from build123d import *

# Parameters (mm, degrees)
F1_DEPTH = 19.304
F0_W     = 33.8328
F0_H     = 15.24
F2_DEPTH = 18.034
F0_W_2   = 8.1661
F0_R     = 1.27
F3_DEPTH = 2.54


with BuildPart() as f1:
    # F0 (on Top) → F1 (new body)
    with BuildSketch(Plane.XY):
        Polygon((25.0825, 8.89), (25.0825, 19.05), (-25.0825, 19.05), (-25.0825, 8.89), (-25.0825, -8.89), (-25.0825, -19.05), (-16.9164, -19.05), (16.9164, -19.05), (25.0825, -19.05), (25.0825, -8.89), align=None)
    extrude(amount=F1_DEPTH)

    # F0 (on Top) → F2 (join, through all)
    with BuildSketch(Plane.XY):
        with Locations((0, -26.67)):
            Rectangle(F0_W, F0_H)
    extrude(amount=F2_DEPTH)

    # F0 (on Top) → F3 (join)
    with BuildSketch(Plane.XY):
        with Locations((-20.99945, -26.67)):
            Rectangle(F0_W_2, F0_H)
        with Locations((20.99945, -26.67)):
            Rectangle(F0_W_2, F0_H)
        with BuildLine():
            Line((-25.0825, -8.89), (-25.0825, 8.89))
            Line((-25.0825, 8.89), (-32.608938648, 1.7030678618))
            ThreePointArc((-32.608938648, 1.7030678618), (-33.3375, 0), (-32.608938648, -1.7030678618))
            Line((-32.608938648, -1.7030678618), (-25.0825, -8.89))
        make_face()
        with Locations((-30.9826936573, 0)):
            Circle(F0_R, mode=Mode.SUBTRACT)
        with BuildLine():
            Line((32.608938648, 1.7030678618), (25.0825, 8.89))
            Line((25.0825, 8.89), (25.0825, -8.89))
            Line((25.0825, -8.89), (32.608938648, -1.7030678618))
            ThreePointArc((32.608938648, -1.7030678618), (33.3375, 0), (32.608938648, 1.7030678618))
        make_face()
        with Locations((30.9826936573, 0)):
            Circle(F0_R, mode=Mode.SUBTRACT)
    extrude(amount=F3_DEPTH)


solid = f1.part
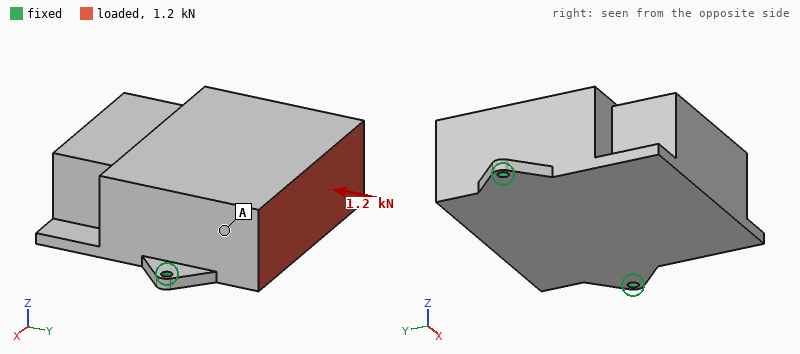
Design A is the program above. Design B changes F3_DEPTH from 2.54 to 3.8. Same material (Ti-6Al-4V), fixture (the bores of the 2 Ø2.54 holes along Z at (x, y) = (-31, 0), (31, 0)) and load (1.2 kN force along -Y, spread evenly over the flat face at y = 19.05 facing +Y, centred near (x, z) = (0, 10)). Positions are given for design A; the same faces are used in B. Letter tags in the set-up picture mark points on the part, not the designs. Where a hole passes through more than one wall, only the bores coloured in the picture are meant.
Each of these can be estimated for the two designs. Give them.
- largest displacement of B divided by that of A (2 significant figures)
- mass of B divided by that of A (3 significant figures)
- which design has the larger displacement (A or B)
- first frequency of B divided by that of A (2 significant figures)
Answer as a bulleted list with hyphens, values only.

- 0.36
- 1.01
- A
- 1.6
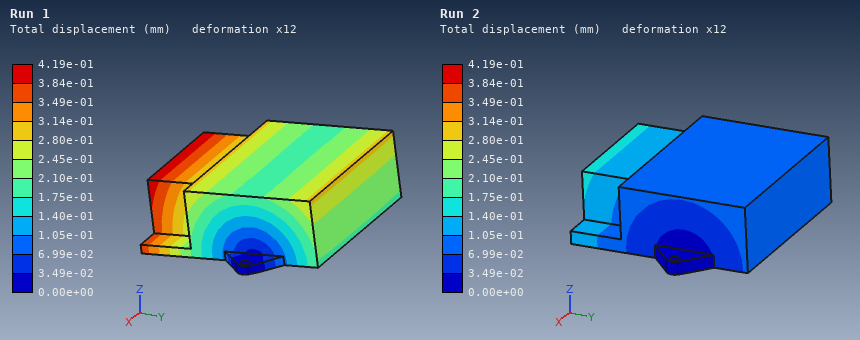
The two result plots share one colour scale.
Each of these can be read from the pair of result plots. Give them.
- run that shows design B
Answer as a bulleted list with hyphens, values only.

- Run 2
